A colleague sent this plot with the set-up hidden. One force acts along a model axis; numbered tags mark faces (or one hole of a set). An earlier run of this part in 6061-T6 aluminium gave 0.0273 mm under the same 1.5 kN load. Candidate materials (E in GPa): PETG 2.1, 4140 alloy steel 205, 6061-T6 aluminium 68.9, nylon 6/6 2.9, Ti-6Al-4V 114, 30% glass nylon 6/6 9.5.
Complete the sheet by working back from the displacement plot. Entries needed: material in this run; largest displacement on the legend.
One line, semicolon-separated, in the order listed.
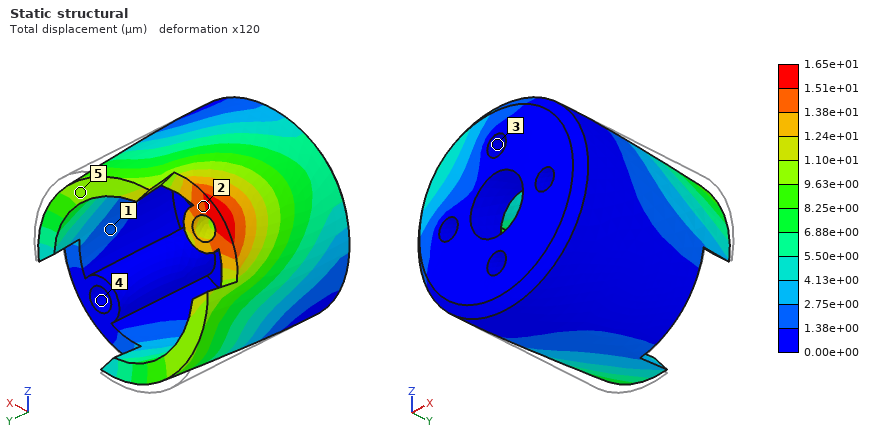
Ti-6Al-4V; 1.65e+01 µm
